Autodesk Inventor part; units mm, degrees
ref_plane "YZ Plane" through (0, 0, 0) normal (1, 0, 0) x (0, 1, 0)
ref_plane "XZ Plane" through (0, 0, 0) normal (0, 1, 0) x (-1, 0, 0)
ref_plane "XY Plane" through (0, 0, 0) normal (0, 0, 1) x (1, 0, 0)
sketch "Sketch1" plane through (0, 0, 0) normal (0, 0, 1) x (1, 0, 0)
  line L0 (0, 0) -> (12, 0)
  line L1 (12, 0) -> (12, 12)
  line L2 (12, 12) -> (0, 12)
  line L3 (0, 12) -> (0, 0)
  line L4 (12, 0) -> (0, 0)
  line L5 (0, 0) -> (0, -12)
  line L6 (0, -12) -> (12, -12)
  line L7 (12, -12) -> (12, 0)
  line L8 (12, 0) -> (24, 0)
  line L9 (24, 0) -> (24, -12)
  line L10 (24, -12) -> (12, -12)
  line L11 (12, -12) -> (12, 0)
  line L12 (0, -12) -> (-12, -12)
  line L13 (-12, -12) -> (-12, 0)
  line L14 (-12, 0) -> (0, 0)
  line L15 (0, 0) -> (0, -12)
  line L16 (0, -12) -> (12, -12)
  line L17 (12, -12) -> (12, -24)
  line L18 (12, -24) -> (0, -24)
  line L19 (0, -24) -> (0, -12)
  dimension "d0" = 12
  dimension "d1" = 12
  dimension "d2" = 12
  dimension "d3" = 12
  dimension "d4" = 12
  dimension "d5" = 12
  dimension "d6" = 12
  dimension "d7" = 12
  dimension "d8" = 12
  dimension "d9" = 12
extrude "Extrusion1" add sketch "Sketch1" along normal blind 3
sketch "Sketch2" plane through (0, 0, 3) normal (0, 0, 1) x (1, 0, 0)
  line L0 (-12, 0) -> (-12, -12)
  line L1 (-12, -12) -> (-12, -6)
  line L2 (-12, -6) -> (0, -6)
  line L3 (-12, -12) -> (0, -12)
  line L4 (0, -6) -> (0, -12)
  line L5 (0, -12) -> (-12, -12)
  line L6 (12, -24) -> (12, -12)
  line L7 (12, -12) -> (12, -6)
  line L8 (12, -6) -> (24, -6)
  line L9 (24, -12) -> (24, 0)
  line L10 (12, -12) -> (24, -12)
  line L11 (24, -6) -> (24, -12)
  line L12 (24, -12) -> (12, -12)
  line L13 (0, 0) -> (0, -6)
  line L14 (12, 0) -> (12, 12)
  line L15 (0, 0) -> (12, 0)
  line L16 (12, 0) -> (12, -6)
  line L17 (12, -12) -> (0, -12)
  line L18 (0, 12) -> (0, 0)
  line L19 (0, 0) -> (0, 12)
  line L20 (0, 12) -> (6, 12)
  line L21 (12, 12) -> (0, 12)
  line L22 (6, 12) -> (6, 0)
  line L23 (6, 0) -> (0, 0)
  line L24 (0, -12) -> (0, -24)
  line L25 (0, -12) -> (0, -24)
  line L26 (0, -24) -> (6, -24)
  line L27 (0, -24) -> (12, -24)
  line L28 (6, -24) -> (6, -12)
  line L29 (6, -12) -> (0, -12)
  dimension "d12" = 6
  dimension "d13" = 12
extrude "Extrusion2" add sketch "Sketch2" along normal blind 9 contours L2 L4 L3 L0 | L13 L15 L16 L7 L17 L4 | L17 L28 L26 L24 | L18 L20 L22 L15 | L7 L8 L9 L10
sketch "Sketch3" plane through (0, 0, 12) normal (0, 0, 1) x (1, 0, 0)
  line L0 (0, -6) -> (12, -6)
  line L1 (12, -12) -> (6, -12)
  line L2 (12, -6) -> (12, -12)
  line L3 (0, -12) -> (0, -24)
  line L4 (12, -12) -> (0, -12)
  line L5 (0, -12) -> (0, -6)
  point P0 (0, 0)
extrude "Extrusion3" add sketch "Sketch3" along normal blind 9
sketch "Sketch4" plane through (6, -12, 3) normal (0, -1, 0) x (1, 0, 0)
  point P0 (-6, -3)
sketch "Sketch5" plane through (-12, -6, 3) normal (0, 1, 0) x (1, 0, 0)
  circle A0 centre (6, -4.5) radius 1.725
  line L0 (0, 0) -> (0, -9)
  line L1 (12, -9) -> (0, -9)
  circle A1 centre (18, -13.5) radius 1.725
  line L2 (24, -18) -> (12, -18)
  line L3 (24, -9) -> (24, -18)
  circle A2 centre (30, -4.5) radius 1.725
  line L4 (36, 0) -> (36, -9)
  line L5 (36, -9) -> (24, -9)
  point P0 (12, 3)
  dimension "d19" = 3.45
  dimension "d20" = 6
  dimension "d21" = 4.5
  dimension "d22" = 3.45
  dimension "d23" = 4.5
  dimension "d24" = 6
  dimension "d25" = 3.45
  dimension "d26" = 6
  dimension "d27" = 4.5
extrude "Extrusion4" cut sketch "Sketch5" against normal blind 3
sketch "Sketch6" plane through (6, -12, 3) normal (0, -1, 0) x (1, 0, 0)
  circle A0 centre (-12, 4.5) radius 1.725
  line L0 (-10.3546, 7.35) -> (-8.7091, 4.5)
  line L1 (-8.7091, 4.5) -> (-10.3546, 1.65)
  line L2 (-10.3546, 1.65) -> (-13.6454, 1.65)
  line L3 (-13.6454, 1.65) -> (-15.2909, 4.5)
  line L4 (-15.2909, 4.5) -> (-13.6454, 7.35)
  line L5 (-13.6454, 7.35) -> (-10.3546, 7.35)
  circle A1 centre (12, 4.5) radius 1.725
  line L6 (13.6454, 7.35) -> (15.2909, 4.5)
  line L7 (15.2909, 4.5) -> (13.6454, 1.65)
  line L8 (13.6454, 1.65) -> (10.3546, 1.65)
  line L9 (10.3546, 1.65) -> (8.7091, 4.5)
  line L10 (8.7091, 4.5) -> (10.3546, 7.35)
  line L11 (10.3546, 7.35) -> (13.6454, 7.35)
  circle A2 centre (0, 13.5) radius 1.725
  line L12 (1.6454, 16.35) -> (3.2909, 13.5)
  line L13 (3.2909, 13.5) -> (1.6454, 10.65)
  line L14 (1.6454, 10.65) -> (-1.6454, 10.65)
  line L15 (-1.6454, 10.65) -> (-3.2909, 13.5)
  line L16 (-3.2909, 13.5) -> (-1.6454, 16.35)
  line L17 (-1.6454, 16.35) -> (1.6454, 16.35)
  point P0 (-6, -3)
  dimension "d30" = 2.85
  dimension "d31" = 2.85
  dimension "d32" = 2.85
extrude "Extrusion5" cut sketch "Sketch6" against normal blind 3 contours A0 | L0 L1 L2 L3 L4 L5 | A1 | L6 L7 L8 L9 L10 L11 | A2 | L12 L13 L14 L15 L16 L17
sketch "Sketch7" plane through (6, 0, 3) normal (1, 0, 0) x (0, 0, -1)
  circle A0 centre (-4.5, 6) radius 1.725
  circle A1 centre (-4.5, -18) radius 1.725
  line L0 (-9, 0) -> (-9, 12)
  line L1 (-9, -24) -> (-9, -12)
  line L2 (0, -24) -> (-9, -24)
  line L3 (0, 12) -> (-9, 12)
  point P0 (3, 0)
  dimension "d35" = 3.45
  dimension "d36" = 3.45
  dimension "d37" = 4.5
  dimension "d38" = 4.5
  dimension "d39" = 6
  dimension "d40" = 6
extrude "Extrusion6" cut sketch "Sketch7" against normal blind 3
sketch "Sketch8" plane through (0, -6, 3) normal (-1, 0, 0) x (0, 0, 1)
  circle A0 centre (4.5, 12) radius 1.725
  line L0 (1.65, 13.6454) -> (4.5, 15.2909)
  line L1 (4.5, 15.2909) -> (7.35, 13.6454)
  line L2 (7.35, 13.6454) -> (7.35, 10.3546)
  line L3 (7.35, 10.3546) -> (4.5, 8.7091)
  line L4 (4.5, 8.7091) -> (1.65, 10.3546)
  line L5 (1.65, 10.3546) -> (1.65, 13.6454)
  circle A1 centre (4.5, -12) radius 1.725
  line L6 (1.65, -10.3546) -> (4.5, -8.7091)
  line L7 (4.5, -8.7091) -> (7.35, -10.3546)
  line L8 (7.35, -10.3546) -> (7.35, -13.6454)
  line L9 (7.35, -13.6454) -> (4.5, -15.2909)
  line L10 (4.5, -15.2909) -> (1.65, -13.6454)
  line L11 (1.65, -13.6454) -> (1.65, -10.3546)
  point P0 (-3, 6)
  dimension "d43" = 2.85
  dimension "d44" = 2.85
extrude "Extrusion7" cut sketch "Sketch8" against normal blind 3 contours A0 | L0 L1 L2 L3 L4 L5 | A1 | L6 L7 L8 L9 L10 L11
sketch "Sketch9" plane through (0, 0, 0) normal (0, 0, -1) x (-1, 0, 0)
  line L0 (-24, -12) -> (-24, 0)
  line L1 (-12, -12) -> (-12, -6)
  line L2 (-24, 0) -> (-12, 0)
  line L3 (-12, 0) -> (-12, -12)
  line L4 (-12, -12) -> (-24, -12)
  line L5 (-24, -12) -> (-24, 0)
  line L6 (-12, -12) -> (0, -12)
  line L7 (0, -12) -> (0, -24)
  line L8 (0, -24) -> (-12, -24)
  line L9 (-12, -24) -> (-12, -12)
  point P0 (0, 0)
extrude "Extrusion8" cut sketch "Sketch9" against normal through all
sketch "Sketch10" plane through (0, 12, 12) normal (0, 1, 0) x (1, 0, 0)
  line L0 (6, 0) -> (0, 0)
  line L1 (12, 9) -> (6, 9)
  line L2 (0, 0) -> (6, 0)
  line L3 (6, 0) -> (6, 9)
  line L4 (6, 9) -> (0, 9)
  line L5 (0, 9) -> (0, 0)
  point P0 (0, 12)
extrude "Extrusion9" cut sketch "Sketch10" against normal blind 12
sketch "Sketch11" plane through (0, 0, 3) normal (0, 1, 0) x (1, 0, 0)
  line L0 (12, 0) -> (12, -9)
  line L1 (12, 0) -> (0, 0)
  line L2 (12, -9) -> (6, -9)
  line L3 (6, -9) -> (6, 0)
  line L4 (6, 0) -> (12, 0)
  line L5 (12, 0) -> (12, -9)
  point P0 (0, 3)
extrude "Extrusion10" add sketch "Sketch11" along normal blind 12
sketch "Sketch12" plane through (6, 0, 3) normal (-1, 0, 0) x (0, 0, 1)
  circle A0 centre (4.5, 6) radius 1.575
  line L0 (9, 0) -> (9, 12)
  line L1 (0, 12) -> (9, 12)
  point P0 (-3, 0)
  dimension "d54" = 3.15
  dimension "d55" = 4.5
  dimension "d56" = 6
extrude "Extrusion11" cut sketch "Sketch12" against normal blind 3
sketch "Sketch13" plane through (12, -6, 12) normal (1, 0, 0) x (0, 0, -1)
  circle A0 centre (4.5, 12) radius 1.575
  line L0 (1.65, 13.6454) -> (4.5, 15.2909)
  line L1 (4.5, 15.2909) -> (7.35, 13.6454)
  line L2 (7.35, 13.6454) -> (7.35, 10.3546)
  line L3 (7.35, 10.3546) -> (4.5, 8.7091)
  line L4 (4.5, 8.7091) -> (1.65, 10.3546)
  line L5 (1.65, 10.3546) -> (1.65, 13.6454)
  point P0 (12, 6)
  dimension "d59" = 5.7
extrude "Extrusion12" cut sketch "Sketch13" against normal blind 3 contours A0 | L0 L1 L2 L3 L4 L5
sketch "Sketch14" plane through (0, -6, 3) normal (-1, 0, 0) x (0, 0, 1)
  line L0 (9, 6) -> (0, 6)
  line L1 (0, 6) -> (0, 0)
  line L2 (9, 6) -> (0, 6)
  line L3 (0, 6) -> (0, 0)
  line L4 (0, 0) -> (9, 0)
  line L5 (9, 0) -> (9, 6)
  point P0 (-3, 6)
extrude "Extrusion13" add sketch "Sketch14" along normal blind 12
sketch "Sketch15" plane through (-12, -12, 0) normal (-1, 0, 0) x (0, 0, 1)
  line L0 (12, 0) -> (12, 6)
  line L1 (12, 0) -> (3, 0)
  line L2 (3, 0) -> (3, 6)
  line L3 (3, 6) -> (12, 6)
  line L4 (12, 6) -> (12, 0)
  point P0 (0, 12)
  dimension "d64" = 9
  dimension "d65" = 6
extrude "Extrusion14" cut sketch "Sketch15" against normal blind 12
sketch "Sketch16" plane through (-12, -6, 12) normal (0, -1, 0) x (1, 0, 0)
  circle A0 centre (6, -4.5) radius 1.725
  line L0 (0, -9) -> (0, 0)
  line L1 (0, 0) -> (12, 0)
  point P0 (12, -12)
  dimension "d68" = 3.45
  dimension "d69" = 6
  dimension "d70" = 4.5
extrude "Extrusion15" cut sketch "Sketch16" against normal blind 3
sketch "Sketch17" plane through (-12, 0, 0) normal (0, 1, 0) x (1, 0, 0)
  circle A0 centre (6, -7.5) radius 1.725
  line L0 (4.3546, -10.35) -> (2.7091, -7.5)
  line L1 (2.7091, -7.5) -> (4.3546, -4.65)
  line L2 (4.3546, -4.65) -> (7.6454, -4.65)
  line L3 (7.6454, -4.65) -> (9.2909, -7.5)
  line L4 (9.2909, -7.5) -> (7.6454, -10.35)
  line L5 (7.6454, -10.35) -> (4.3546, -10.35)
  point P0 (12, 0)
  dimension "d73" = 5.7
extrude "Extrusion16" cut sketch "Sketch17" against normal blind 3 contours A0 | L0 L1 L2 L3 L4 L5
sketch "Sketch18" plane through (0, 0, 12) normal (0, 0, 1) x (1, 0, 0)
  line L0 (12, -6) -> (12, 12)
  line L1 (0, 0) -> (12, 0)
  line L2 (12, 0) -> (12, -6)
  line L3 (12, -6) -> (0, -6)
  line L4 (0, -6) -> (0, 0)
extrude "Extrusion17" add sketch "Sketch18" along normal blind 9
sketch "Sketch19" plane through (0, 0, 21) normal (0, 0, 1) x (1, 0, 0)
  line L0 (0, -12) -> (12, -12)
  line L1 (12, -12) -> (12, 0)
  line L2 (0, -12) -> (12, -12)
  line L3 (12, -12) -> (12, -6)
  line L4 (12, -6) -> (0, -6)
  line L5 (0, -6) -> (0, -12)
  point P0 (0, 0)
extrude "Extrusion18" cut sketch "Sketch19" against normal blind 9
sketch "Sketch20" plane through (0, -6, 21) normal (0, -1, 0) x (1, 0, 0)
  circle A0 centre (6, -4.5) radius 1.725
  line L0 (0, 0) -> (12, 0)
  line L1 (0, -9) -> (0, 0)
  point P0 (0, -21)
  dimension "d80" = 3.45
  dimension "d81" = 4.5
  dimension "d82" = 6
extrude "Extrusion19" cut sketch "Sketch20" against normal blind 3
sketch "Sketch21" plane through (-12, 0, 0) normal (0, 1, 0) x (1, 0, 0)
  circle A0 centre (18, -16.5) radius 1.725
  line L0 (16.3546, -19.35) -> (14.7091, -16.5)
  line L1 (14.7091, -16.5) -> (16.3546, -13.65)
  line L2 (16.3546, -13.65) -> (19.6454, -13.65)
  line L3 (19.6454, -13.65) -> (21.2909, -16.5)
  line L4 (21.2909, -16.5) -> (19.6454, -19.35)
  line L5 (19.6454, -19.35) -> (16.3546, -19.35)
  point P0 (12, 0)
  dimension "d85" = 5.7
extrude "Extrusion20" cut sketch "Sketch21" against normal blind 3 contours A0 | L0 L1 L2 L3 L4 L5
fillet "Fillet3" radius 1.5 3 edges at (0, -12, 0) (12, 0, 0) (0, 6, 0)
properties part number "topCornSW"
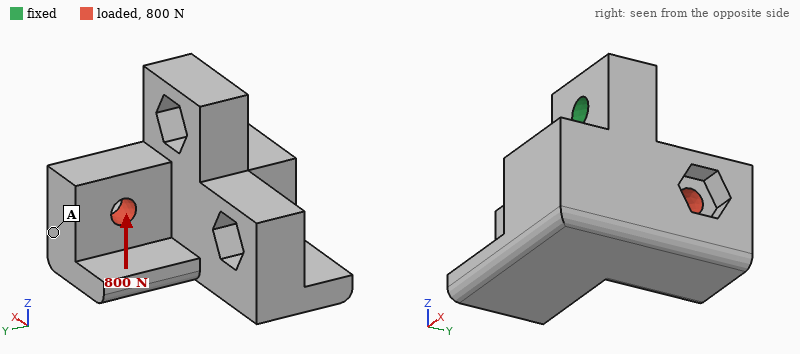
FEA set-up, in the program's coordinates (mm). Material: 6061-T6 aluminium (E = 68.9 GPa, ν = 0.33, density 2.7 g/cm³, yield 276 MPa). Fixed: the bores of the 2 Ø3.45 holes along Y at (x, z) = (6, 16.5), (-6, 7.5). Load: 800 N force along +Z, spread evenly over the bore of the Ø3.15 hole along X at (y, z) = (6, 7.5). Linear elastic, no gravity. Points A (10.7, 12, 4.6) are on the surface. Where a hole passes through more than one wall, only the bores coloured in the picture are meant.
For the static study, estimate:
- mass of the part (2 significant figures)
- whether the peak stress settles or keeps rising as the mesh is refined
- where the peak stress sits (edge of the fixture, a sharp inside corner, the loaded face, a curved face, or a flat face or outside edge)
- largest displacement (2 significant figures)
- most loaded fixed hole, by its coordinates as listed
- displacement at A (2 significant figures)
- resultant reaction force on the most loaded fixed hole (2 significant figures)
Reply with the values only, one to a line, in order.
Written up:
11 g
keeps rising
edge of the fixture
82 µm
(6, 16.5)
72 µm
830 N
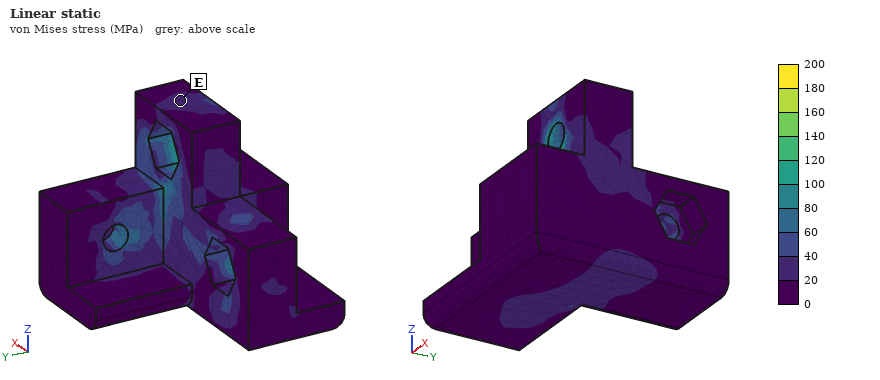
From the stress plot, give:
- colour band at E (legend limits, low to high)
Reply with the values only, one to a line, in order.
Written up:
20 to 40 MPa
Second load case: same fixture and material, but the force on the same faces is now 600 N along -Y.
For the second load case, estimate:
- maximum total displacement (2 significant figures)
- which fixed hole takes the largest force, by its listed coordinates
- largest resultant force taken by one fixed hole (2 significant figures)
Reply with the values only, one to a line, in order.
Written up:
39 µm
(6, 16.5)
420 N
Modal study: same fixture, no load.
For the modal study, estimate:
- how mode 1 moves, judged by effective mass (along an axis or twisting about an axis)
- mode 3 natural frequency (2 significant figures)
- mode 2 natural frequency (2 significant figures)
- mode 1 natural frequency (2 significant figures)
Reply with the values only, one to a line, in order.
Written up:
along Y
27 kHz
19 kHz
7500 Hz
